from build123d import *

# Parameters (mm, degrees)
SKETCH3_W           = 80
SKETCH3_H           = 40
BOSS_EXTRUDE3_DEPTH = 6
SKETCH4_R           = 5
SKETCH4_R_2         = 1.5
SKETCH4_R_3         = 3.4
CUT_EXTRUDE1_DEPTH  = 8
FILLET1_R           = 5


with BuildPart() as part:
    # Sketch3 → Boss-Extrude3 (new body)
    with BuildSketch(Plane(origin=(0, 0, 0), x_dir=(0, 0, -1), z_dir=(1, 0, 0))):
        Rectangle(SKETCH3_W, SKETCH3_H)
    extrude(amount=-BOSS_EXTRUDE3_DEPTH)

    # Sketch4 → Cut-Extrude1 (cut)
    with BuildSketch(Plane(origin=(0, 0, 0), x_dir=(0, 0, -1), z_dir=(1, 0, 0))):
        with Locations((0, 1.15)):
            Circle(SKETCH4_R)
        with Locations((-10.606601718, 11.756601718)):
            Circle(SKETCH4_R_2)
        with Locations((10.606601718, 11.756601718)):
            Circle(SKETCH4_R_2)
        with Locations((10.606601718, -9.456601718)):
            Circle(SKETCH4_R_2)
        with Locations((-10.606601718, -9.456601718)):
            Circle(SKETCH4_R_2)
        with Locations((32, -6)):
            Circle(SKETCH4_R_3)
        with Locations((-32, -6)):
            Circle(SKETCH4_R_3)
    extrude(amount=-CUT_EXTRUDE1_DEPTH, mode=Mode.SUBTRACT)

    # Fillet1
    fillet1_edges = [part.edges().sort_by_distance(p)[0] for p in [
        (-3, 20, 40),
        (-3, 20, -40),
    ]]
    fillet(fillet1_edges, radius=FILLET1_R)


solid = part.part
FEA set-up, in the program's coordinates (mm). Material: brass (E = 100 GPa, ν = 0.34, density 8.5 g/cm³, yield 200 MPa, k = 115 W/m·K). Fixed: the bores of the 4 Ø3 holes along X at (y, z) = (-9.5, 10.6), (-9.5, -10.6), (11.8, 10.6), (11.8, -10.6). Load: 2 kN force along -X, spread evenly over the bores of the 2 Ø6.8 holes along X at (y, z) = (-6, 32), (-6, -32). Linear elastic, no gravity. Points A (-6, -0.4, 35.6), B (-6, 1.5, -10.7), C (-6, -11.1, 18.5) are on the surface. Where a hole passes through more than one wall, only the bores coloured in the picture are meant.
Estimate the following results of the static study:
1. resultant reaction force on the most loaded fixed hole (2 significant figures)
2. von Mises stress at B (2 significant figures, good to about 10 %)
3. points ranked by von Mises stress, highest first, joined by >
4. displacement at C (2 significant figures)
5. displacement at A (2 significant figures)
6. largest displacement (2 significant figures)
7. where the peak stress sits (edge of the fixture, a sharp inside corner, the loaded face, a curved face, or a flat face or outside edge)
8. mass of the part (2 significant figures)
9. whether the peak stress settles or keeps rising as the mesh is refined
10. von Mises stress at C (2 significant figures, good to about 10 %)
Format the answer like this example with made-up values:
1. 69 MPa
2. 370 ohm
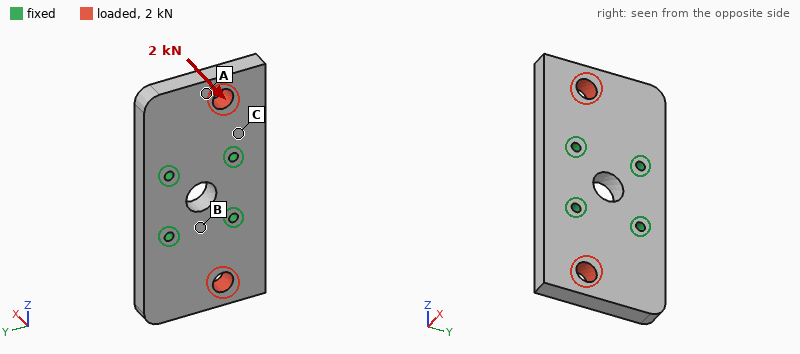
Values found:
1. 780 N
2. 38 MPa
3. C > B > A
4. 0.018 mm
5. 0.076 mm
6. 0.10 mm
7. edge of the fixture
8. 150 g
9. keeps rising
10. 63 MPa
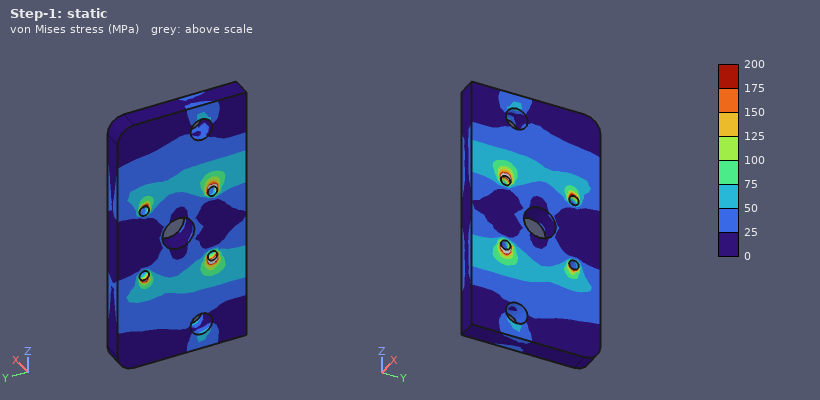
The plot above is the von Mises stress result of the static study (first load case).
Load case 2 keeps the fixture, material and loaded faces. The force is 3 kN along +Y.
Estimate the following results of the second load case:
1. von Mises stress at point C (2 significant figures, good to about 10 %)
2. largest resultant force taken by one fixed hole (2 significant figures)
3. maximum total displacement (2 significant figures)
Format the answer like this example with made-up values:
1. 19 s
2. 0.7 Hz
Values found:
1. 12 MPa
2. 1.1 kN
3. 10 µm
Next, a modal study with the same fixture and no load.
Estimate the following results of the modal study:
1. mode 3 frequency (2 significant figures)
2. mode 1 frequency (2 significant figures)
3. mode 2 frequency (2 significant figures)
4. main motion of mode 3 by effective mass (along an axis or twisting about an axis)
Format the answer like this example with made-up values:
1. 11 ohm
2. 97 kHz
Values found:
1. 6400 Hz
2. 3600 Hz
3. 3600 Hz
4. twisting about Z
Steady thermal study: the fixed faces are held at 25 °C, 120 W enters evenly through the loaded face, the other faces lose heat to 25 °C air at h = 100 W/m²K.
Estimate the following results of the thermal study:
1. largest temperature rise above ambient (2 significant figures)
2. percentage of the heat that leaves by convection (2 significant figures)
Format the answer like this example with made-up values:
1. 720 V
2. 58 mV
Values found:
1. 68 K
2. 15 %
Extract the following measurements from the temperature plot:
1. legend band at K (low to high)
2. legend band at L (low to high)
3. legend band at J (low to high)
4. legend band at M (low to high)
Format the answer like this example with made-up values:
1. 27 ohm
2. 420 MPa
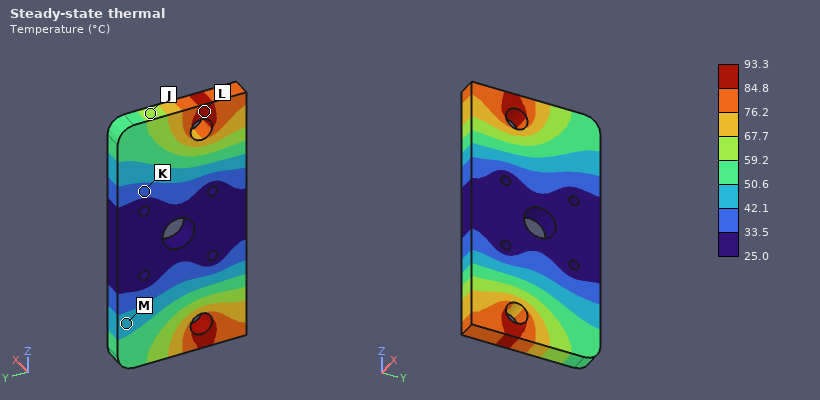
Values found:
1. 33.5 to 42.1 °C
2. 84.8 to 93.3 °C
3. 59.2 to 67.7 °C
4. 42.1 to 50.6 °C
